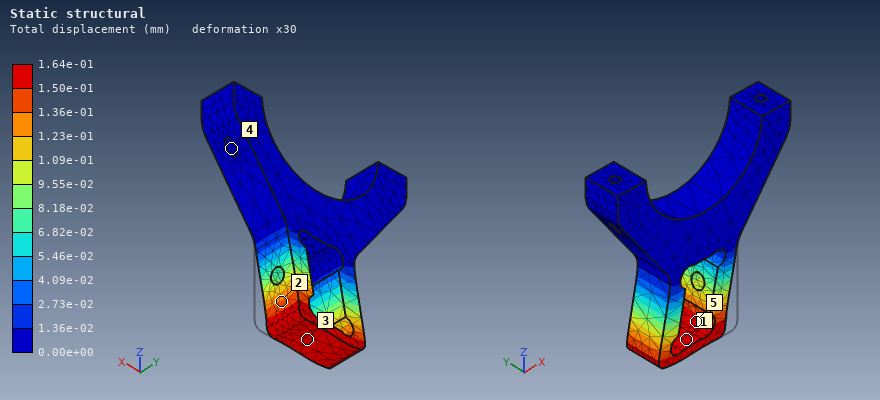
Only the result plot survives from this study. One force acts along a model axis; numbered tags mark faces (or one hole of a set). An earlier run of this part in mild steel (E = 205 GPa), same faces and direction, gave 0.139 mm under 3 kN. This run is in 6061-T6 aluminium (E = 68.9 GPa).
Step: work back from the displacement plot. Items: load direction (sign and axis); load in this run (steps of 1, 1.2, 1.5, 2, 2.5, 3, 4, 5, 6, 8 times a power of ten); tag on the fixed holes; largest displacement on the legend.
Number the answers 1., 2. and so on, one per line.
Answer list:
1. -X
2. 1.2 kN
3. 4
4. 1.64e-01 mm
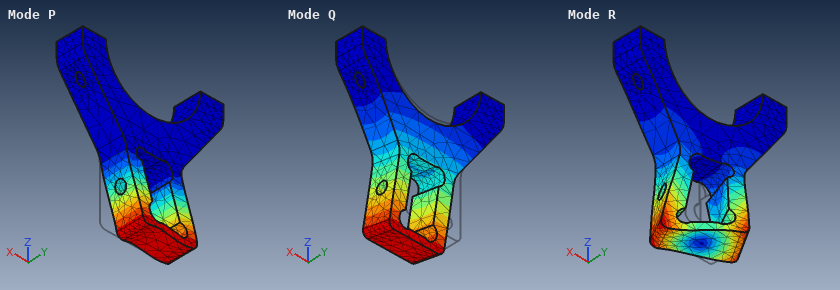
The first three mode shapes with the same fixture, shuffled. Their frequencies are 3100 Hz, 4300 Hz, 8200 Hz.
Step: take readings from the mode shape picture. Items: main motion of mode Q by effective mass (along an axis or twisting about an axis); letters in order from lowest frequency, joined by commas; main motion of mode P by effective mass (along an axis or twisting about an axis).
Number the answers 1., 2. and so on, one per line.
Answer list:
1. along Y
2. Q, P, R
3. along X
